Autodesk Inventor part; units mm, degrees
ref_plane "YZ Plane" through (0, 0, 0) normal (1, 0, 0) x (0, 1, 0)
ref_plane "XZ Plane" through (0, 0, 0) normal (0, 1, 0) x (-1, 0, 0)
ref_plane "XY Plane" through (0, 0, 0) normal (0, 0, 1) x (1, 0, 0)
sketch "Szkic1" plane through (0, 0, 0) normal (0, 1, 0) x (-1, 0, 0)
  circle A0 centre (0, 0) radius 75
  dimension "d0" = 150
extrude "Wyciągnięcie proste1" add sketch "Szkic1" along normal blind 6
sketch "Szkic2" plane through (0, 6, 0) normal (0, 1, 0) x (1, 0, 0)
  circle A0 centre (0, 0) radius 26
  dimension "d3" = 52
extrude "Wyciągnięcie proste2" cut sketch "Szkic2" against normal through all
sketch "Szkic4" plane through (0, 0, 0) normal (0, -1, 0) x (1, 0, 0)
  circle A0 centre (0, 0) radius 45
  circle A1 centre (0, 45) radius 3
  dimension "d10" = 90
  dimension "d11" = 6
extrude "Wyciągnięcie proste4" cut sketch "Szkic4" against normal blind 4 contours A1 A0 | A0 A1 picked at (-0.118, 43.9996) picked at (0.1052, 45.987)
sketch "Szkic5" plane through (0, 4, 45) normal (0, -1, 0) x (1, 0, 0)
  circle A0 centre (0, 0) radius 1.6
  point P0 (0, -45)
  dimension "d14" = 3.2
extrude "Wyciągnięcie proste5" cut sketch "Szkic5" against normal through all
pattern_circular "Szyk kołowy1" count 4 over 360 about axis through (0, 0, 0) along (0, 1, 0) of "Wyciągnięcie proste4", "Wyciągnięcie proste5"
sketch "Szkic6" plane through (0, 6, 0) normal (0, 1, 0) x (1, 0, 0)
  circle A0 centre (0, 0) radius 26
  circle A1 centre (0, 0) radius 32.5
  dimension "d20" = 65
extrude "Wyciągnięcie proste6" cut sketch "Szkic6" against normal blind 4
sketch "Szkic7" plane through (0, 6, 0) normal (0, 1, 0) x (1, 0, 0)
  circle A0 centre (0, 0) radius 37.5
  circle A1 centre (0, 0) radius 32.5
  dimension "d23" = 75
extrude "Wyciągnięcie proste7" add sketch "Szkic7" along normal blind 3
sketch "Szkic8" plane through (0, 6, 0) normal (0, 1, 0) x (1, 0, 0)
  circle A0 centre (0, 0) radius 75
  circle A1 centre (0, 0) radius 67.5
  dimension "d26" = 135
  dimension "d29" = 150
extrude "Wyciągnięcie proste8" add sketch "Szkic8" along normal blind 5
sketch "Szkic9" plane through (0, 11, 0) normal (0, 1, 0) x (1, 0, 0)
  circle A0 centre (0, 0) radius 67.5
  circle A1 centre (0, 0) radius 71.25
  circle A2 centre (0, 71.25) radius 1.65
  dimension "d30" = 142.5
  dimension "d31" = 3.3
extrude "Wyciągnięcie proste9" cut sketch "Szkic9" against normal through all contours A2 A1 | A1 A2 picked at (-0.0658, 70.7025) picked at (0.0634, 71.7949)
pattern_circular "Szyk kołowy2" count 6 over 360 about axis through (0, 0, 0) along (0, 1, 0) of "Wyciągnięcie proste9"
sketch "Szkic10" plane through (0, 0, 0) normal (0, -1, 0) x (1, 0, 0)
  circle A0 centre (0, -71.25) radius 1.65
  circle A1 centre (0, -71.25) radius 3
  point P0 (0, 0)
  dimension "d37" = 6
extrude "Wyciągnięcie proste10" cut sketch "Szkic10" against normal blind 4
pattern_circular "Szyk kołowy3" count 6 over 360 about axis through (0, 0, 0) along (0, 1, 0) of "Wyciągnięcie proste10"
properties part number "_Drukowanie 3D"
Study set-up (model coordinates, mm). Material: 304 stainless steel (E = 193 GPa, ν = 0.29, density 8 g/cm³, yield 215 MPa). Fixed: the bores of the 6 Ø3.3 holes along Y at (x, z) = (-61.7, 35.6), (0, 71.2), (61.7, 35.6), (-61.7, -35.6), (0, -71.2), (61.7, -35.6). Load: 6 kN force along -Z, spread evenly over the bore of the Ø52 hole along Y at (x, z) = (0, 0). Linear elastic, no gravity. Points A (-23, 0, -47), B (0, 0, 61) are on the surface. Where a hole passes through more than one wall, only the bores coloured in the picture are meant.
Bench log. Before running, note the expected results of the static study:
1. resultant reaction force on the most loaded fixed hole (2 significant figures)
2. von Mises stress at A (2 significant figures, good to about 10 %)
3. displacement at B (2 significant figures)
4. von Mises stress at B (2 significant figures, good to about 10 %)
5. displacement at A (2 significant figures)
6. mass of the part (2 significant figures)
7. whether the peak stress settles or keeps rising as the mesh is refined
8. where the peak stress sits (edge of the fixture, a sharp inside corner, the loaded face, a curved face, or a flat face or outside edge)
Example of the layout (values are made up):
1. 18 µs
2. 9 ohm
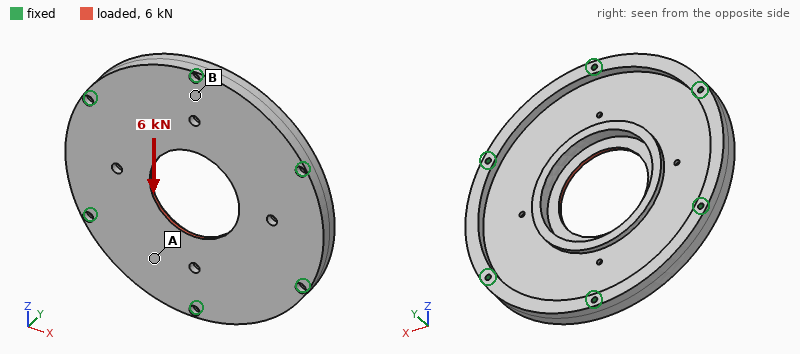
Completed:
1. 1.2 kN
2. 4.1 MPa
3. 2.3 µm
4. 10.0 MPa
5. 2.8 µm
6. 860 g
7. keeps rising
8. edge of the fixture
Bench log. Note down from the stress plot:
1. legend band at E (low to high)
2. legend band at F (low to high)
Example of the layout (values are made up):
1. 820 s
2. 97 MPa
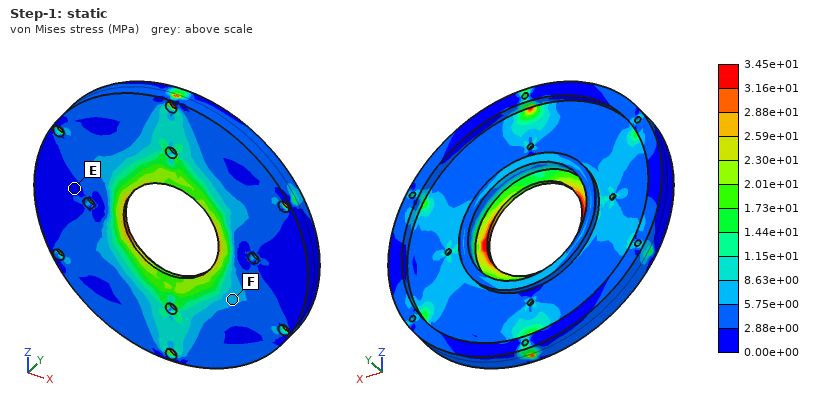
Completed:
1. 0.00e+00 to 2.88e+00 MPa
2. 5.75e+00 to 8.63e+00 MPa
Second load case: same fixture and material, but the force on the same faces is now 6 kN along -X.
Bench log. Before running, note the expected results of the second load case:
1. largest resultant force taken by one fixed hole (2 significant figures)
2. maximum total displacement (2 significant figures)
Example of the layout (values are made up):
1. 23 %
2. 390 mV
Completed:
1. 1.1 kN
2. 7.9 µm
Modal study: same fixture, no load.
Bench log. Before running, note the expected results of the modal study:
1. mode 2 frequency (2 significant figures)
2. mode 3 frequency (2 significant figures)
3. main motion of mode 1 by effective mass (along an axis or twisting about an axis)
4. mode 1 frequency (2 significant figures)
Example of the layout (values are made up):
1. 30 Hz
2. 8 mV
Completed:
1. 4100 Hz
2. 4100 Hz
3. along Y
4. 2800 Hz
